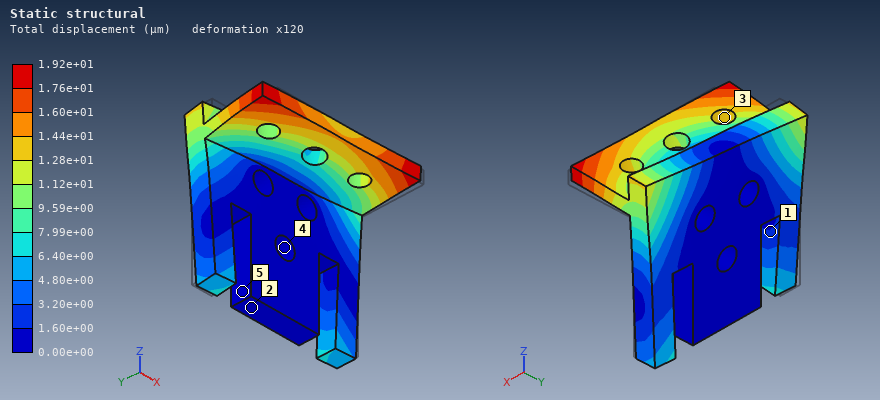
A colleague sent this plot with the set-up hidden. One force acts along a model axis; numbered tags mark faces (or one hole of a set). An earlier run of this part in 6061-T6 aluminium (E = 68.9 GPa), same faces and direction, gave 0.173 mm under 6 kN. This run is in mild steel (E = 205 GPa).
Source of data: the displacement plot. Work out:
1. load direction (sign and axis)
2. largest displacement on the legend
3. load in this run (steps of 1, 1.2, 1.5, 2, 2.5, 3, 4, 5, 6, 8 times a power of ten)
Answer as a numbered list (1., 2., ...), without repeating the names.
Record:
1. -X
2. 1.92e+01 µm
3. 2 kN
